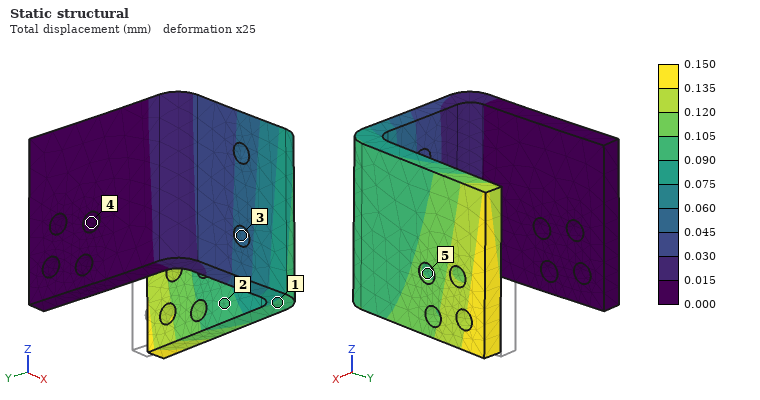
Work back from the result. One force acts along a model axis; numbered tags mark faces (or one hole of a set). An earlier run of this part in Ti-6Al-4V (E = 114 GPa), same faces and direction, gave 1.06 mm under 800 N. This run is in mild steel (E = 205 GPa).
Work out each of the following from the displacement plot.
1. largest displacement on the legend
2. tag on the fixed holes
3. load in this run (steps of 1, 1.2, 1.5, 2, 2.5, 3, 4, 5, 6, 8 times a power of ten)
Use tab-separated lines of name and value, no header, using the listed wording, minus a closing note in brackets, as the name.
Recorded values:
largest displacement on the legend	0.150 mm
tag on the fixed holes	4
load in this run	200 N
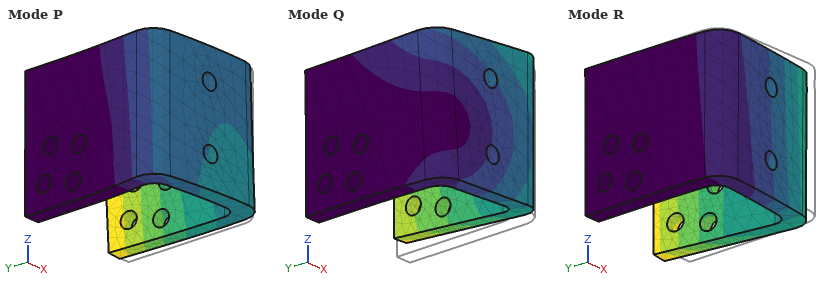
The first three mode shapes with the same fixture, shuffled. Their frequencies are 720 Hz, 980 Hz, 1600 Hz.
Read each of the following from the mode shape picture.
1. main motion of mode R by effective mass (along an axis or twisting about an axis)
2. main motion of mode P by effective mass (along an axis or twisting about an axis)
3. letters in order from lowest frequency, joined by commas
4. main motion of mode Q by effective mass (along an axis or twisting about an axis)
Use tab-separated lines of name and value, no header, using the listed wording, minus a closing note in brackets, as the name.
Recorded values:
main motion of mode R by effective mass	along Y
main motion of mode P by effective mass	along X
letters in order from lowest frequency, joined by commas	R, Q, P
main motion of mode Q by effective mass	along Z
